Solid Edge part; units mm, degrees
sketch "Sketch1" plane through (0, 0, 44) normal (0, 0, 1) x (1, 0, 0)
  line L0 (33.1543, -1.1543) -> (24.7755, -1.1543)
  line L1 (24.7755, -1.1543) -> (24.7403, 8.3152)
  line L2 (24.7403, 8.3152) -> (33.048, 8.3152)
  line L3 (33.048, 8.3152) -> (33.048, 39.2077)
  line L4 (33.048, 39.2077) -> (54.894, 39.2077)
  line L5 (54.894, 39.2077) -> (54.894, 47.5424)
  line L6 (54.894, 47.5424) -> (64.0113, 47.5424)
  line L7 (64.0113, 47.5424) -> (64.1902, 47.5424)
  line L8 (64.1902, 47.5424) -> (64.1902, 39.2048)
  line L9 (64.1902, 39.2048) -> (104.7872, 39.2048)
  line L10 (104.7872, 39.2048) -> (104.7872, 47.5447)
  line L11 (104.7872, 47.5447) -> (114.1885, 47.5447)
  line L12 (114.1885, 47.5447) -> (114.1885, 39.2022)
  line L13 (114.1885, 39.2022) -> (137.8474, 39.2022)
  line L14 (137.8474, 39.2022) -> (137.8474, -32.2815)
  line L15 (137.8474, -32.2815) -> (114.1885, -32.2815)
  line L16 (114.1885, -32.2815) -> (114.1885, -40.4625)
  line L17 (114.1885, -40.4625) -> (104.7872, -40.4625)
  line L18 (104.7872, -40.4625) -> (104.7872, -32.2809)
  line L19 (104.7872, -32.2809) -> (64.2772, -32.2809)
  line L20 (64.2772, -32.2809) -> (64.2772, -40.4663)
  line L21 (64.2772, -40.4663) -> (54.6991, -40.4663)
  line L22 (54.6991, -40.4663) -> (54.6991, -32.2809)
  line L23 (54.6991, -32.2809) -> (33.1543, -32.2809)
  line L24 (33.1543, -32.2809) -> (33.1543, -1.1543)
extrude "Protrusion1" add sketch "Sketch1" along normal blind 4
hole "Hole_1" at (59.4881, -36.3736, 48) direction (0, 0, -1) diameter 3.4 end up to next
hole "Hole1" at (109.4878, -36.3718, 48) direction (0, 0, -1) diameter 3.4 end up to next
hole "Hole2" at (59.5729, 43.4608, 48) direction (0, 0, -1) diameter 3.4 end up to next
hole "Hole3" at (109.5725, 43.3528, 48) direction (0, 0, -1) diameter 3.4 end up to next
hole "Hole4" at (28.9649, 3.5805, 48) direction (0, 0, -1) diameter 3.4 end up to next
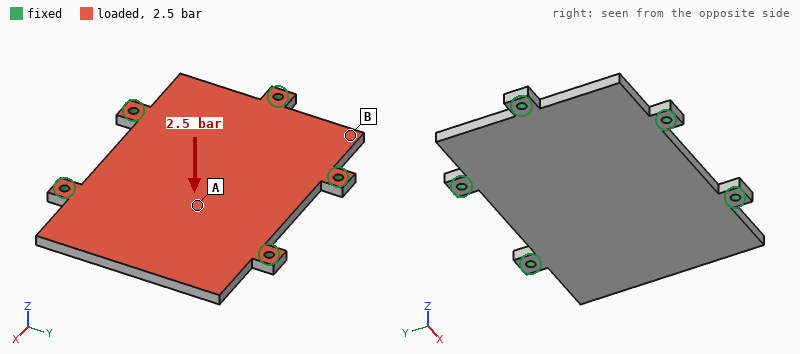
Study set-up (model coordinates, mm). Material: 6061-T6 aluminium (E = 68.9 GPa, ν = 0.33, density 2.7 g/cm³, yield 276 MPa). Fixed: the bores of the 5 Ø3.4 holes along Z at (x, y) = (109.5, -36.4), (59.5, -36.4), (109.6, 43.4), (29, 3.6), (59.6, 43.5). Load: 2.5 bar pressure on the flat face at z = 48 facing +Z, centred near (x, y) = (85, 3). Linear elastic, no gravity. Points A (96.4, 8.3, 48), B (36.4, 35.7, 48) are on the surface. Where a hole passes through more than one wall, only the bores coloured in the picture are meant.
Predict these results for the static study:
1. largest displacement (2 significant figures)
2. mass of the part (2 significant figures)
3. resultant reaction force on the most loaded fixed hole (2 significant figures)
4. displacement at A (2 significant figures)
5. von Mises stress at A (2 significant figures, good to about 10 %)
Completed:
0.27 mm
85 g
540 N
0.13 mm
32 MPa
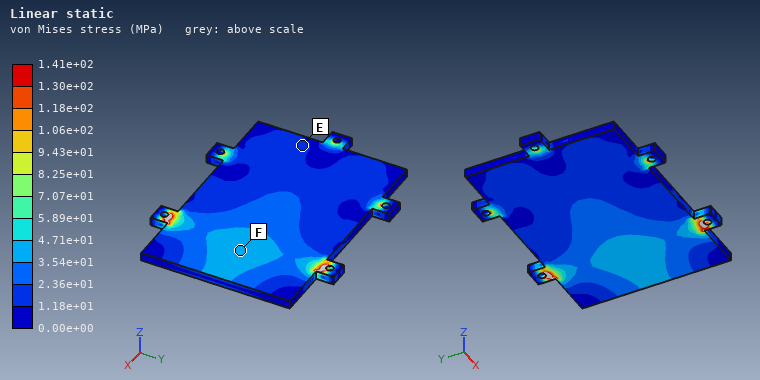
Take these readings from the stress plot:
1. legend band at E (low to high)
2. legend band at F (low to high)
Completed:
1.18e+01 to 2.36e+01 MPa
3.54e+01 to 4.71e+01 MPa
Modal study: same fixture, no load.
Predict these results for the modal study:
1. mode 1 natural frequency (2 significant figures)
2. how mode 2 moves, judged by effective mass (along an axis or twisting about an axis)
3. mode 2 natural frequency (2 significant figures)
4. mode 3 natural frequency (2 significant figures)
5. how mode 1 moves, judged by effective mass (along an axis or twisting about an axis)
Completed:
1900 Hz
along Z
2900 Hz
4400 Hz
along Z
